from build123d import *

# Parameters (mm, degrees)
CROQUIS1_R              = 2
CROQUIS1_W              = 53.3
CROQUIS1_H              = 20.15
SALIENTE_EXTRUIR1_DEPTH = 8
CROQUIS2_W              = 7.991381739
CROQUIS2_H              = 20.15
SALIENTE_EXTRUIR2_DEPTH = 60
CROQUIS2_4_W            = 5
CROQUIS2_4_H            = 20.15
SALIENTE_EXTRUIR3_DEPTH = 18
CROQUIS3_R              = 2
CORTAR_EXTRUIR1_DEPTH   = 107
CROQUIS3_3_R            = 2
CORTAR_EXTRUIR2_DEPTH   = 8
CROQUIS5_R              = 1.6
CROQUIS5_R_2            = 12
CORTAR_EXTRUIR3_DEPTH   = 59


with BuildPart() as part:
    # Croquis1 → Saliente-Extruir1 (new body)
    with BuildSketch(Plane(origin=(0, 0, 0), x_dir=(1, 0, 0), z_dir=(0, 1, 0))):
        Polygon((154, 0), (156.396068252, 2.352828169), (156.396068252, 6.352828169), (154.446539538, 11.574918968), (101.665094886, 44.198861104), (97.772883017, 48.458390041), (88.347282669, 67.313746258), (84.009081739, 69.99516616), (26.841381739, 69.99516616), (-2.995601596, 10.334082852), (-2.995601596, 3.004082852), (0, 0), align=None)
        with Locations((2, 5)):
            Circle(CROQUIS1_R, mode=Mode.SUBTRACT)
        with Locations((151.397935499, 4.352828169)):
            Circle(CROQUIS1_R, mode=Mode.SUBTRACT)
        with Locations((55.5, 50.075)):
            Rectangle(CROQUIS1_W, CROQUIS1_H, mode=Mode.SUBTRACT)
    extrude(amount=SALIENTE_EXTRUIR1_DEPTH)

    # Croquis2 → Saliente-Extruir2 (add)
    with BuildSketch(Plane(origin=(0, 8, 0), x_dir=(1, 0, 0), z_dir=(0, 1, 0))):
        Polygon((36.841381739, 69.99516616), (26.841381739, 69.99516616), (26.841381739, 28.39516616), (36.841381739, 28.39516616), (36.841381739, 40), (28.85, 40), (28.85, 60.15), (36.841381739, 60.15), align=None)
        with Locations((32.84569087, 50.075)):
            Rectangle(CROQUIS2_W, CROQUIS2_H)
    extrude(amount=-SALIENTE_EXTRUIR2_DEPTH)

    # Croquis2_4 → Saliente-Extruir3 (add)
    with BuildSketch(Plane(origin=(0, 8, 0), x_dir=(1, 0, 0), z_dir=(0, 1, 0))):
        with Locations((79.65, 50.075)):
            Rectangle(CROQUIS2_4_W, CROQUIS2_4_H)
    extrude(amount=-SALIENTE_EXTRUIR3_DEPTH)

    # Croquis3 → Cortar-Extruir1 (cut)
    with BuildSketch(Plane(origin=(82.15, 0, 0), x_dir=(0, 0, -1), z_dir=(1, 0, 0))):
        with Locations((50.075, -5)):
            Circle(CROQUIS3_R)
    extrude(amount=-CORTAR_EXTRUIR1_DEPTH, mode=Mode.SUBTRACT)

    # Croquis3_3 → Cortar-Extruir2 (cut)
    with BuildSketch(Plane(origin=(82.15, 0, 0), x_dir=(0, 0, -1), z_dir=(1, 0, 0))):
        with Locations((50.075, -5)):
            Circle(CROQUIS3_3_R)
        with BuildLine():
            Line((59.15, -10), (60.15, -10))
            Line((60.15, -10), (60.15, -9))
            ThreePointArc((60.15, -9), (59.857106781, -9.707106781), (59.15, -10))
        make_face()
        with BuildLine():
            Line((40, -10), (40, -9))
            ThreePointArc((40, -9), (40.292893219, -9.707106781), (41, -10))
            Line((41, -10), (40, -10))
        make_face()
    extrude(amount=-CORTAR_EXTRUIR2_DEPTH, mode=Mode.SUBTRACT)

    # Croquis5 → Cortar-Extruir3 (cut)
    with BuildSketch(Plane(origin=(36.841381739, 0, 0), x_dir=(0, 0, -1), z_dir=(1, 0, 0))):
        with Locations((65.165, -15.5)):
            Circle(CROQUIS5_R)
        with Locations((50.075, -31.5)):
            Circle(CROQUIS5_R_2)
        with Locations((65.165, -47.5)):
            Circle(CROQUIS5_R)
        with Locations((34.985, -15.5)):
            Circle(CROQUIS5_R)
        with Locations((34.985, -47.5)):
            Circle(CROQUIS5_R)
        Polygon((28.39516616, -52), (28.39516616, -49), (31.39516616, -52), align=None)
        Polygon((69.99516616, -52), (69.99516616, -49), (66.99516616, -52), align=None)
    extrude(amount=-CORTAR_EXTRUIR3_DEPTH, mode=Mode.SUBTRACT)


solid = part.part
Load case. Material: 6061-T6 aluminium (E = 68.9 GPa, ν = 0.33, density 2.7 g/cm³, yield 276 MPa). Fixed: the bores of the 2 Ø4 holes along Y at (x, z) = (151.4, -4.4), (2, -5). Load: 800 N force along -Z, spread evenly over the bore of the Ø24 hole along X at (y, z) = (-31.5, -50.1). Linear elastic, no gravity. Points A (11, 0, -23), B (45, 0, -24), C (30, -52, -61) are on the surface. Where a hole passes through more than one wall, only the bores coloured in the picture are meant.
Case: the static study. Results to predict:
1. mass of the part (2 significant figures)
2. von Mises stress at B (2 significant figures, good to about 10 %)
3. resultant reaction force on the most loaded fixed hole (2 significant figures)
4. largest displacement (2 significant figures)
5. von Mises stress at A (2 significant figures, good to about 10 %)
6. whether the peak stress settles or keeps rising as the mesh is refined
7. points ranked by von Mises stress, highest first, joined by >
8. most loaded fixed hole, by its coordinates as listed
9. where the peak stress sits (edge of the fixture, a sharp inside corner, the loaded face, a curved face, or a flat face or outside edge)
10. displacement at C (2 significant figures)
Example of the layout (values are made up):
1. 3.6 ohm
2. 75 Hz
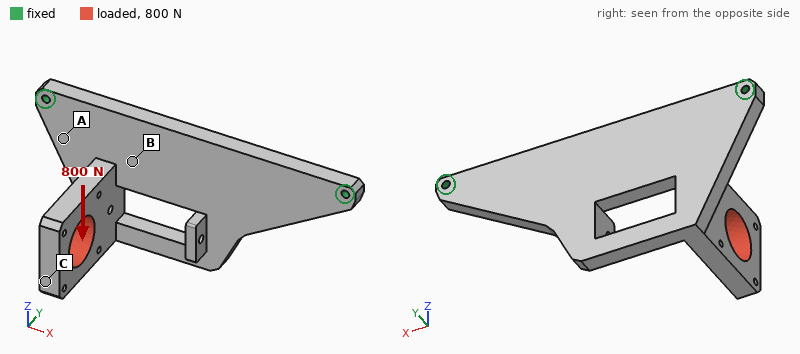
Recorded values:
1. 200 g
2. 19 MPa
3. 720 N
4. 0.73 mm
5. 61 MPa
6. keeps rising
7. A > B > C
8. (2, -5)
9. edge of the fixture
10. 0.69 mm
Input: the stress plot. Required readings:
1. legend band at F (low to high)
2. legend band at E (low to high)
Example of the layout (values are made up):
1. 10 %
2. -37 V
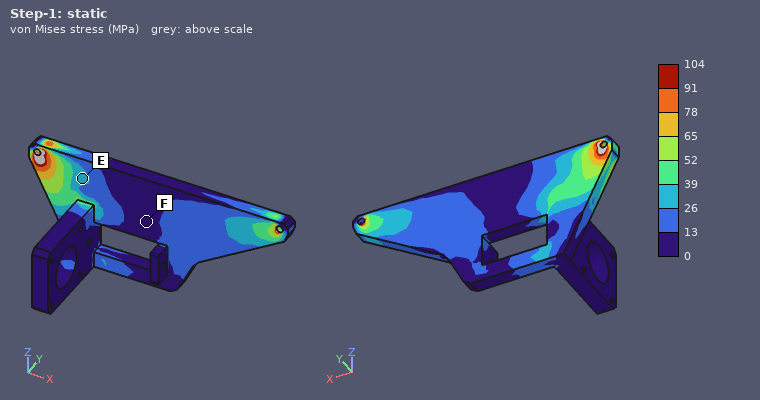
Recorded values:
1. 0 to 13 MPa
2. 26 to 39 MPa
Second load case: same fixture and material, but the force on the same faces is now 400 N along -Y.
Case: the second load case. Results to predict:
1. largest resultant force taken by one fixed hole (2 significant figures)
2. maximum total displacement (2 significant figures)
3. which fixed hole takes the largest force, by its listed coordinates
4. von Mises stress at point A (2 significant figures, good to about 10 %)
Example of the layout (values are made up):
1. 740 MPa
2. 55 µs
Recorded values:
1. 340 N
2. 0.38 mm
3. (2, -5)
4. 27 MPa
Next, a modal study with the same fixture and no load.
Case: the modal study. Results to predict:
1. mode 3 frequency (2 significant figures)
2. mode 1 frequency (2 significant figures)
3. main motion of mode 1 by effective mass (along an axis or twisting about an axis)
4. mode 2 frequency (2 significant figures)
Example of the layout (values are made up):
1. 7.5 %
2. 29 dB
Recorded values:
1. 2100 Hz
2. 610 Hz
3. along Y
4. 1200 Hz
